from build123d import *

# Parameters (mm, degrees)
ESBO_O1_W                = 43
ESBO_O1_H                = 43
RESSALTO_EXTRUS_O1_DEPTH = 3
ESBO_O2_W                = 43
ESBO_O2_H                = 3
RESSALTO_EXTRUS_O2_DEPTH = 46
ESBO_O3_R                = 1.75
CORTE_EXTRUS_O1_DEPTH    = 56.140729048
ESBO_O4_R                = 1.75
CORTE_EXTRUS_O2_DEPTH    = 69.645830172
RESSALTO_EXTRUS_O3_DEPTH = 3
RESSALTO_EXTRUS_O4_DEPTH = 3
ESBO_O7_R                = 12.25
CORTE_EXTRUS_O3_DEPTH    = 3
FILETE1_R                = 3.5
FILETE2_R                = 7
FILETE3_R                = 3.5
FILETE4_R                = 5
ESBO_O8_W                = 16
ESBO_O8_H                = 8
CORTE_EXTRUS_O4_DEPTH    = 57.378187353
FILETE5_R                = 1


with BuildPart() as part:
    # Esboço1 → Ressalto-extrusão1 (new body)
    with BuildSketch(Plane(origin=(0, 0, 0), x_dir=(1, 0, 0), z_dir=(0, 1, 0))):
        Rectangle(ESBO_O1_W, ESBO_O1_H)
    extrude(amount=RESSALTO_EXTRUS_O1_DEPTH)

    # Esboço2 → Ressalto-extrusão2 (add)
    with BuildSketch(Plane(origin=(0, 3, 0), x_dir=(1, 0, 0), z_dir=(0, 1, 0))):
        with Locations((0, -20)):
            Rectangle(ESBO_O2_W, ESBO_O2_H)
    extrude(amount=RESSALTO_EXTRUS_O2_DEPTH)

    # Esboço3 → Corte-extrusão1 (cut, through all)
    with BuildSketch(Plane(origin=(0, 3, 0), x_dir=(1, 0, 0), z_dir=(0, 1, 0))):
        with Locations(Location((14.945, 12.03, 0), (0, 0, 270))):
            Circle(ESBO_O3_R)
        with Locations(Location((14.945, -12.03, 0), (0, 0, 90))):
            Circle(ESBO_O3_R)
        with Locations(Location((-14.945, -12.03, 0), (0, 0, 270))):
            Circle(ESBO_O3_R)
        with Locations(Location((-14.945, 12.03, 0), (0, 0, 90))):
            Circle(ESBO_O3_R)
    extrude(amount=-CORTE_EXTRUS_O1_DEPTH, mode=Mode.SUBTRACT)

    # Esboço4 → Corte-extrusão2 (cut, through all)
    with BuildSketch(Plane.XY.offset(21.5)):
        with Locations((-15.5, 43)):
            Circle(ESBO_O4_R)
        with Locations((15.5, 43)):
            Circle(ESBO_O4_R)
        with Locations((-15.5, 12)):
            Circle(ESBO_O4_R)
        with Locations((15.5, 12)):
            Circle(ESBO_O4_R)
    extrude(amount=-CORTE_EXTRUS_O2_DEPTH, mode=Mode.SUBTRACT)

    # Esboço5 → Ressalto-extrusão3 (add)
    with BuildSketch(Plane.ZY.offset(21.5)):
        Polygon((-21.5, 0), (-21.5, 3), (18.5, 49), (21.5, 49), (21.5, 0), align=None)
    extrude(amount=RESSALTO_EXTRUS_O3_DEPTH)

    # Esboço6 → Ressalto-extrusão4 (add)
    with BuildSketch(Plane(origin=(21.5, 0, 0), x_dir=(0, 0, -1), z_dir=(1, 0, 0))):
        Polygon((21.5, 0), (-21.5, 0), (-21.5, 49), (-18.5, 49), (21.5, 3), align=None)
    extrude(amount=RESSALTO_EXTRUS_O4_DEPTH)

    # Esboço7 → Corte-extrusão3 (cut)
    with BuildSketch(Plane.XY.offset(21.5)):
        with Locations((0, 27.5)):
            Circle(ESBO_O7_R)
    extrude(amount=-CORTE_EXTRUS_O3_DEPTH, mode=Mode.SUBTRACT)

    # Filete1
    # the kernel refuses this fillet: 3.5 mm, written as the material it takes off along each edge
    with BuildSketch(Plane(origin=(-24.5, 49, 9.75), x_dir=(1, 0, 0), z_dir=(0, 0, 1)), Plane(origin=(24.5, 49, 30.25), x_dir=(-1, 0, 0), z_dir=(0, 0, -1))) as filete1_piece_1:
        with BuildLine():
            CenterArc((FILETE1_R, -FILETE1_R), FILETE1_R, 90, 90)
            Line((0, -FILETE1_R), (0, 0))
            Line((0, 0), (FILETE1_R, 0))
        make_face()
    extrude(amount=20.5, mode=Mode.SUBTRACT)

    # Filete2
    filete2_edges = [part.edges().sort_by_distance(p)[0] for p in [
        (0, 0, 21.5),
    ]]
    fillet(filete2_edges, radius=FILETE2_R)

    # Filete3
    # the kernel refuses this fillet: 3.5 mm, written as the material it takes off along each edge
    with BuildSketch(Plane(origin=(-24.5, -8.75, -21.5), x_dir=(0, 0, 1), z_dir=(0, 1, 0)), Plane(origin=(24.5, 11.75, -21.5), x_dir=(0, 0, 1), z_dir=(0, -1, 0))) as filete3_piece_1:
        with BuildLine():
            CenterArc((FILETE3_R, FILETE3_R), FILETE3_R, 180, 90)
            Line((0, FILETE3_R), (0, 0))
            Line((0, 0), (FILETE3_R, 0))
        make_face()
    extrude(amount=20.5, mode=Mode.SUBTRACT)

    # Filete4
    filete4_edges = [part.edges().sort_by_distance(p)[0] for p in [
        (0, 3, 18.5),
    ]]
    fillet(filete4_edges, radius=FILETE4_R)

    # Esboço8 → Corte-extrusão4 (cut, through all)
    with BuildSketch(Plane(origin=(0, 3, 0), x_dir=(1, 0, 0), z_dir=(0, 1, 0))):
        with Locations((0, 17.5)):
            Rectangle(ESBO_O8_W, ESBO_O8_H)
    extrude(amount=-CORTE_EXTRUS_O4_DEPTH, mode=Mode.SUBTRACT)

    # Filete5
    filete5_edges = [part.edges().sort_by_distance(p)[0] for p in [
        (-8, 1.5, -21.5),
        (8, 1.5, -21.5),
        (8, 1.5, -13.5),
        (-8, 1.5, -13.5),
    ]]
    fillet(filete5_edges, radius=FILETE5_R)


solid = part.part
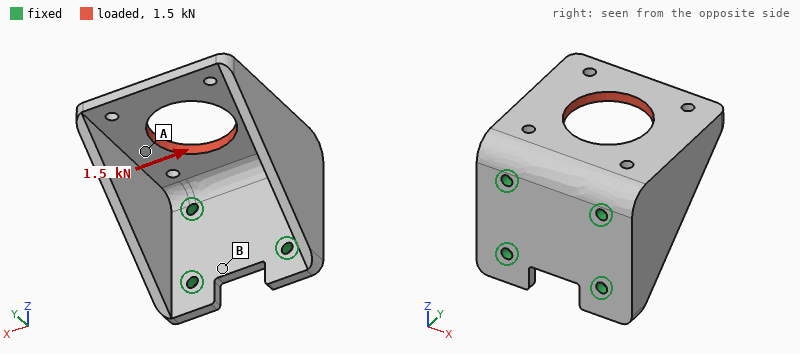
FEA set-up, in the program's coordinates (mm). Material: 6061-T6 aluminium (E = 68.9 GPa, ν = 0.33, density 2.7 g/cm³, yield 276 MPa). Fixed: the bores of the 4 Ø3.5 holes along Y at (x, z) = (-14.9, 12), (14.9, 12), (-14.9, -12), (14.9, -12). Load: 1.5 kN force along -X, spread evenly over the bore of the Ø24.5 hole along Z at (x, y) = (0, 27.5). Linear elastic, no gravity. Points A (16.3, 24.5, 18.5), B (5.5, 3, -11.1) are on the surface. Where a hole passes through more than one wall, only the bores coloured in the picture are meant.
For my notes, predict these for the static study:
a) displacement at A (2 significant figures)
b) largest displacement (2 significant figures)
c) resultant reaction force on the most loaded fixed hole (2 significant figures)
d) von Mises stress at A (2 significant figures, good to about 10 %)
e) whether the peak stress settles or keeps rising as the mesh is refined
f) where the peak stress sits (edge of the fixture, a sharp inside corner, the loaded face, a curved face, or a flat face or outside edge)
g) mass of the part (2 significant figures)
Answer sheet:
0.065 mm
0.13 mm
1.5 kN
32 MPa
keeps rising
edge of the fixture
44 g
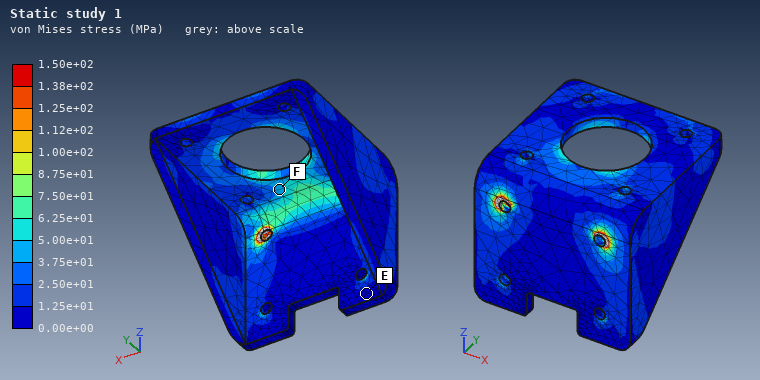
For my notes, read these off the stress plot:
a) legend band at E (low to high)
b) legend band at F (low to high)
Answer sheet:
0.00e+00 to 1.25e+01 MPa
3.75e+01 to 5.00e+01 MPa
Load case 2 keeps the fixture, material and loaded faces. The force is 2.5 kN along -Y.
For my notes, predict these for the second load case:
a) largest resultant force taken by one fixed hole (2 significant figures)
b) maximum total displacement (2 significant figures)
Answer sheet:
1.5 kN
97 µm
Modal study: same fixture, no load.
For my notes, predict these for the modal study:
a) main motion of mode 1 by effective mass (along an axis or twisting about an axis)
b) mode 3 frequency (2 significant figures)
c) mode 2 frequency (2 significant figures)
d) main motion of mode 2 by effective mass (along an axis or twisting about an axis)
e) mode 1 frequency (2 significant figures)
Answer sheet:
along Z
6000 Hz
3900 Hz
along X
3500 Hz
